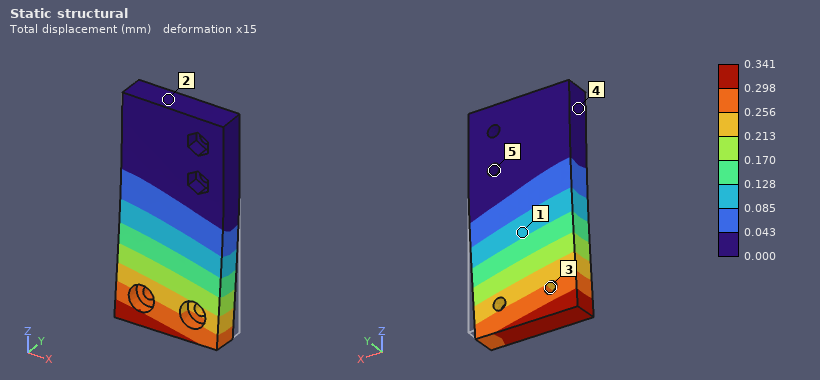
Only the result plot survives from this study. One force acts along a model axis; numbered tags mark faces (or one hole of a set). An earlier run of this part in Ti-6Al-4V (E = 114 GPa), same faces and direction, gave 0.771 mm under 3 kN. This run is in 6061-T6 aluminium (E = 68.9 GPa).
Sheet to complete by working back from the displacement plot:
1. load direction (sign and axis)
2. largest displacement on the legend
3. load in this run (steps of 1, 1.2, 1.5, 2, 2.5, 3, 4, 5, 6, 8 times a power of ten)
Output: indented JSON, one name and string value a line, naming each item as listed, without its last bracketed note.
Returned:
{
  "load direction": "-Y",
  "largest displacement on the legend": "0.341 mm",
  "load in this run": "800 N"
}
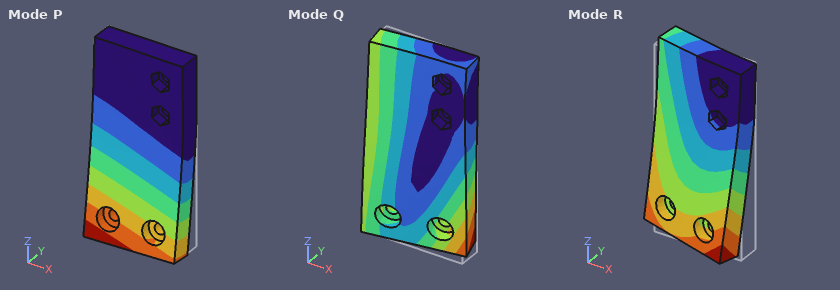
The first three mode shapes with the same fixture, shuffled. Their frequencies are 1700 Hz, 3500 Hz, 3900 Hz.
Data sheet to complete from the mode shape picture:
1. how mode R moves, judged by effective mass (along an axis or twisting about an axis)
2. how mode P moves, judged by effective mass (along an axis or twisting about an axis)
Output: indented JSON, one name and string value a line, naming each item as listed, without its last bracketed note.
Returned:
{
  "how mode R moves, judged by effective mass": "along X",
  "how mode P moves, judged by effective mass": "along Y"
}
